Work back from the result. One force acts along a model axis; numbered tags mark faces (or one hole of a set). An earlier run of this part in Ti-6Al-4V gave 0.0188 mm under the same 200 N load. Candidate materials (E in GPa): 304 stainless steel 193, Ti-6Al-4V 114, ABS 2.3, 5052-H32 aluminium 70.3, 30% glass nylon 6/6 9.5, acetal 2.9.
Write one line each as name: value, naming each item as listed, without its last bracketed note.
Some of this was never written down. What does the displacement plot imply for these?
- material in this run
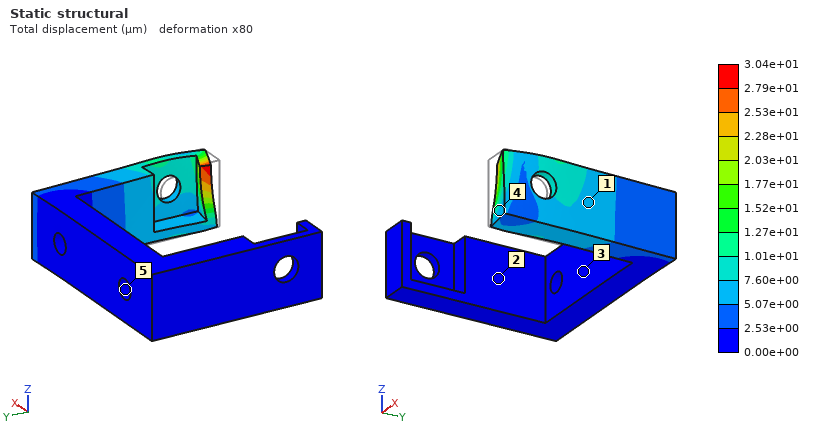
material in this run: 5052-H32 aluminium
